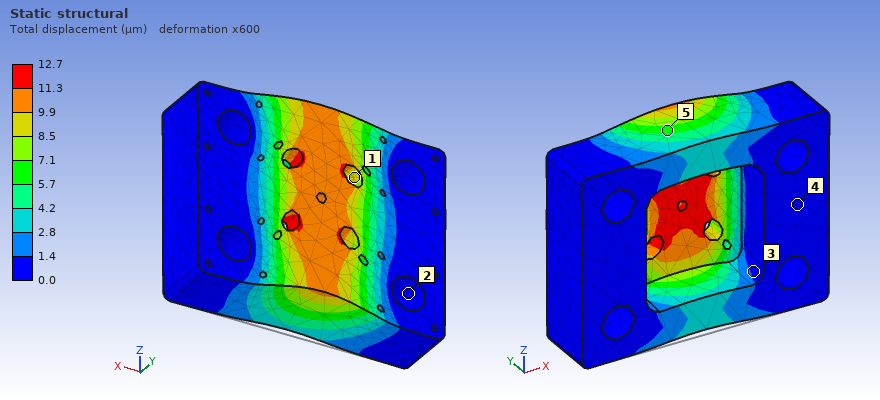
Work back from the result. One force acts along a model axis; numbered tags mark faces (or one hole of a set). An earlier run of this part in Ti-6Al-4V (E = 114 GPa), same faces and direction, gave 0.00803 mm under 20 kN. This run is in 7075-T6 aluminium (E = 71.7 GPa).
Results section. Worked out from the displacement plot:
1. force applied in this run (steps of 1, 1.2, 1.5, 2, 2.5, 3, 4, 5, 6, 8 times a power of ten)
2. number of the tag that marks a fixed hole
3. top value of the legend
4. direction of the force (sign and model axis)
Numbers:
20 kN
2
12.7 µm
+Z
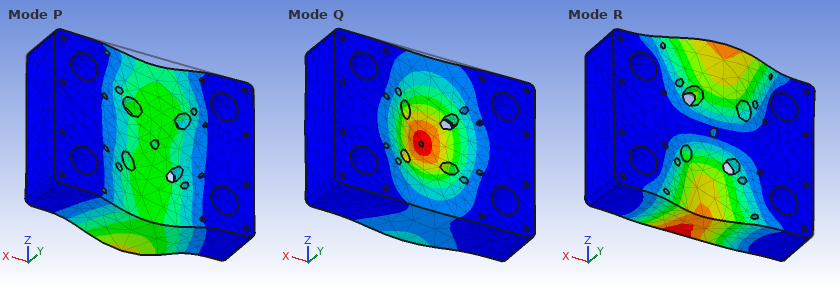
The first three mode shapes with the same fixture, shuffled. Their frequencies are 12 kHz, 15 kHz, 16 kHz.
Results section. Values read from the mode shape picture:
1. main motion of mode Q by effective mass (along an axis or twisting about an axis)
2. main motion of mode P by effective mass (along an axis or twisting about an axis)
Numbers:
along Y
along Z
